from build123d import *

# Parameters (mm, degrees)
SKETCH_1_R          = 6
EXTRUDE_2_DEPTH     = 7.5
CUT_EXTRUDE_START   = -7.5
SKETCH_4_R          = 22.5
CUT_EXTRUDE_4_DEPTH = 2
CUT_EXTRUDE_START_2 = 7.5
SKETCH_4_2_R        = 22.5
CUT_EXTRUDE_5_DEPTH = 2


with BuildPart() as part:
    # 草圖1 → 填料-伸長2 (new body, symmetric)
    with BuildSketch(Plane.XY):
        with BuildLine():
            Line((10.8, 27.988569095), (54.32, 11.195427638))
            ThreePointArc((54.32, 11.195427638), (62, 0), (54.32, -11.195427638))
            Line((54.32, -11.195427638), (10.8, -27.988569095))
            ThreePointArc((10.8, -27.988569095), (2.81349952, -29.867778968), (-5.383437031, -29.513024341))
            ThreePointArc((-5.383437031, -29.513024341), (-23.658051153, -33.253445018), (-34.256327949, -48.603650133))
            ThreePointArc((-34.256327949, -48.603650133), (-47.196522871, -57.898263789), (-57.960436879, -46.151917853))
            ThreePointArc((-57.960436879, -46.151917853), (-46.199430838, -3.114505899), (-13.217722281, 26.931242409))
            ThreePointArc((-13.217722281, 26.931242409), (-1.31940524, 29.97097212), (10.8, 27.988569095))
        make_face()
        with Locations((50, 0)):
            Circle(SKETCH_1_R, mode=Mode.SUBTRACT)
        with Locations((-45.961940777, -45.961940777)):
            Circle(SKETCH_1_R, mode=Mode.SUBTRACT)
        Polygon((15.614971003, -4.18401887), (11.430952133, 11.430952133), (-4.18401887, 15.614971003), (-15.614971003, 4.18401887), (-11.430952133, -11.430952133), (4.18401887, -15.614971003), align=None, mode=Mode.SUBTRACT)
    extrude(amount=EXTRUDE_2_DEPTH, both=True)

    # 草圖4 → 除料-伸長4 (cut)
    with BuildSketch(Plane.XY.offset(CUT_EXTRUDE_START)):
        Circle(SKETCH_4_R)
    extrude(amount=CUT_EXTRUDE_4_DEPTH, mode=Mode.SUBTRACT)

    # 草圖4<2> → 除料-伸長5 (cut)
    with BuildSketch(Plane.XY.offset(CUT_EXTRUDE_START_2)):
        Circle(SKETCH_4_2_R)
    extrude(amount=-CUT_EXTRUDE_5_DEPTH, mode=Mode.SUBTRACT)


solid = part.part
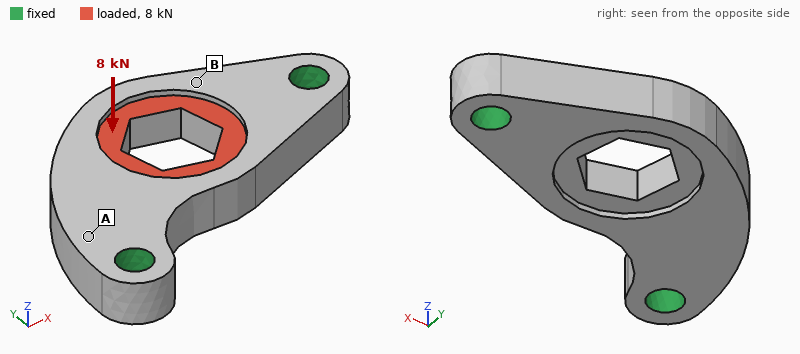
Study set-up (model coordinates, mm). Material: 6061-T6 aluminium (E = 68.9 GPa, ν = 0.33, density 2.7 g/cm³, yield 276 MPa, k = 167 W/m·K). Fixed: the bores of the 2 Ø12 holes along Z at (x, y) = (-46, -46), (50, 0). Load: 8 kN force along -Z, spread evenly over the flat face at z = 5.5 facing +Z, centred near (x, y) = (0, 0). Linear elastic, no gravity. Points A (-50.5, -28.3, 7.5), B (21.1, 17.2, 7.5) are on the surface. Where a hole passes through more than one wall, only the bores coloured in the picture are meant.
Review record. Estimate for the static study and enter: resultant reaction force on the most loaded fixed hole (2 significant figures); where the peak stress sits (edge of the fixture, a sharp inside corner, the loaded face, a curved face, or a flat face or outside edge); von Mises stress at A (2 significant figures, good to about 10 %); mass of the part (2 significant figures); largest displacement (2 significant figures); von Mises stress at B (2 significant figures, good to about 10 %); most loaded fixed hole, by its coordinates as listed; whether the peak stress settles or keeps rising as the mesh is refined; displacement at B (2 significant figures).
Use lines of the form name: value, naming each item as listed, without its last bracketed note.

resultant reaction force on the most loaded fixed hole: 4.9 kN
where the peak stress sits: edge of the fixture
von Mises stress at A: 56 MPa
mass of the part: 180 g
largest displacement: 0.22 mm
von Mises stress at B: 29 MPa
most loaded fixed hole, by its coordinates as listed: (50, 0)
whether the peak stress settles or keeps rising as the mesh is refined: keeps rising
displacement at B: 0.093 mm
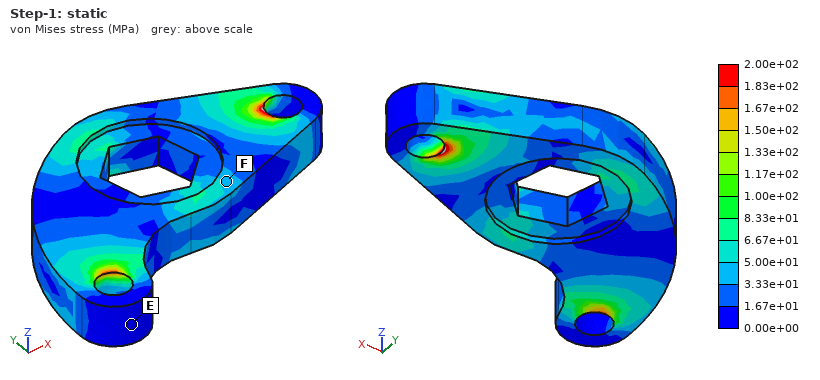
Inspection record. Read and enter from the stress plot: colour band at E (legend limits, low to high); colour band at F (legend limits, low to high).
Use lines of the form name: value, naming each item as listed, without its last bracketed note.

colour band at E: 0.00e+00 to 1.67e+01 MPa
colour band at F: 3.33e+01 to 5.00e+01 MPa
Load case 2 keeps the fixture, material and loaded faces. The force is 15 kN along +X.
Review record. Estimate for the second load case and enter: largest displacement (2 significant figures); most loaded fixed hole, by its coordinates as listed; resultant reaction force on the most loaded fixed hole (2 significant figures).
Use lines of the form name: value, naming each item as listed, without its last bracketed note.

largest displacement: 67 µm
most loaded fixed hole, by its coordinates as listed: (50, 0)
resultant reaction force on the most loaded fixed hole: 11 kN
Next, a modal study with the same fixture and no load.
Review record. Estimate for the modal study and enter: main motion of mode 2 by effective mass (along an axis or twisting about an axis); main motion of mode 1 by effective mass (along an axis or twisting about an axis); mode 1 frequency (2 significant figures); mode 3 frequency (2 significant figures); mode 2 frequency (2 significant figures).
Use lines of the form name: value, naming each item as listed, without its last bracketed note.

main motion of mode 2 by effective mass: along Z
main motion of mode 1 by effective mass: along Z
mode 1 frequency: 3600 Hz
mode 3 frequency: 8900 Hz
mode 2 frequency: 7600 Hz
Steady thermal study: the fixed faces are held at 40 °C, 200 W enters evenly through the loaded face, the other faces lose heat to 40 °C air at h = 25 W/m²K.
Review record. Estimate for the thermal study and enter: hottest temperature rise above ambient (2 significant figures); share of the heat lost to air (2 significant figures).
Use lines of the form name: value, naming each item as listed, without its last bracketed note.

hottest temperature rise above ambient: 60 K
share of the heat lost to air: 5.3 %
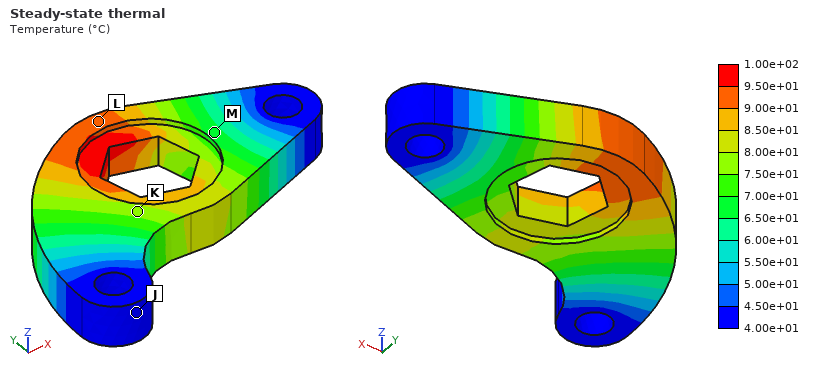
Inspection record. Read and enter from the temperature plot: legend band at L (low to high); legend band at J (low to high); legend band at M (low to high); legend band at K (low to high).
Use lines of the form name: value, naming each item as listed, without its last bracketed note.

legend band at L: 9.00e+01 to 9.50e+01 °C
legend band at J: 4.00e+01 to 4.50e+01 °C
legend band at M: 6.50e+01 to 7.00e+01 °C
legend band at K: 7.50e+01 to 8.00e+01 °C
